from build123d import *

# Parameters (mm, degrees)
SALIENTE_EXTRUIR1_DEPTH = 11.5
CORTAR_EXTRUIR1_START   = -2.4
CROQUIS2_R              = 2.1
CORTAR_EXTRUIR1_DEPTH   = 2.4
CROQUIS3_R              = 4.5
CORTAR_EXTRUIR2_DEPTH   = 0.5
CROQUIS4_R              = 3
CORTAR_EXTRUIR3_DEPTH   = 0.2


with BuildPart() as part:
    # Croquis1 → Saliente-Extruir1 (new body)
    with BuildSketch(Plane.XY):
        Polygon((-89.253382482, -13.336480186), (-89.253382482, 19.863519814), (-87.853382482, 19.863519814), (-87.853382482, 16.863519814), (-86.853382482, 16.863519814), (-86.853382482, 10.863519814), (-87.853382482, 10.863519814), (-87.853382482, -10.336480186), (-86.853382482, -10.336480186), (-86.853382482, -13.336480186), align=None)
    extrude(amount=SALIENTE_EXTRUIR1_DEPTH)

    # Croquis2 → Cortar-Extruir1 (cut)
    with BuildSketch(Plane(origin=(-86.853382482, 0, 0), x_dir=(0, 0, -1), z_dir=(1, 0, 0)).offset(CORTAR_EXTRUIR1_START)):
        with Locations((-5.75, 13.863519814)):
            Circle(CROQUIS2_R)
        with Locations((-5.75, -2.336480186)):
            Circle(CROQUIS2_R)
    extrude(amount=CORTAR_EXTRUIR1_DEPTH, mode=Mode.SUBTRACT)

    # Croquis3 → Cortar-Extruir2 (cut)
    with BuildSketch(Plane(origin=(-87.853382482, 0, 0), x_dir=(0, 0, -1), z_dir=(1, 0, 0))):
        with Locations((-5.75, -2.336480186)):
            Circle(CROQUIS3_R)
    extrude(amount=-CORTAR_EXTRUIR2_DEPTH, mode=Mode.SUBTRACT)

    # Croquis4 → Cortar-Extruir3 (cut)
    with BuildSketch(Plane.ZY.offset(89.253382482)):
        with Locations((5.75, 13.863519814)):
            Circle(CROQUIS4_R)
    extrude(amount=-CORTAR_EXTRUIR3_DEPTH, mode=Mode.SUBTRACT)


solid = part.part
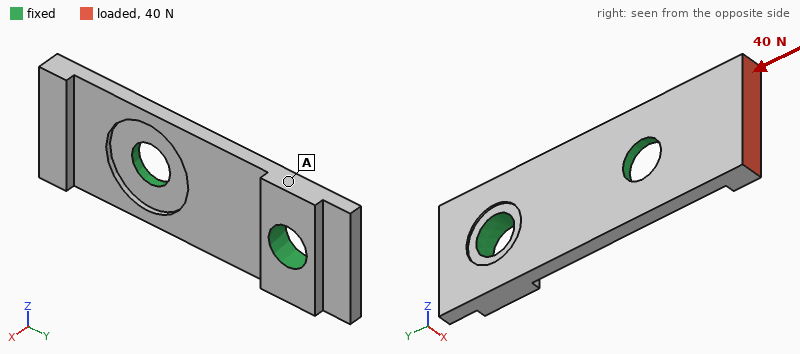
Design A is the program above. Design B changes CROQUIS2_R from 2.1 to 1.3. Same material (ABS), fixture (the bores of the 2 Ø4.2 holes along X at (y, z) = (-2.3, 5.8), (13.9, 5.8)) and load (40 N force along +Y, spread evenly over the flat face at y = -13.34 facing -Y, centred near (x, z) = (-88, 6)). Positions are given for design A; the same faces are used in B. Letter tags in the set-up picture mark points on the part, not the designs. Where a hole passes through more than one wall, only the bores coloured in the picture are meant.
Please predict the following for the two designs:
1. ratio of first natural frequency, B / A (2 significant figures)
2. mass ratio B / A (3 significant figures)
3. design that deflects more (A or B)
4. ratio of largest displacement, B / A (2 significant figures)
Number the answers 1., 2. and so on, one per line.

1. 0.81
2. 1.05
3. B
4. 1.3
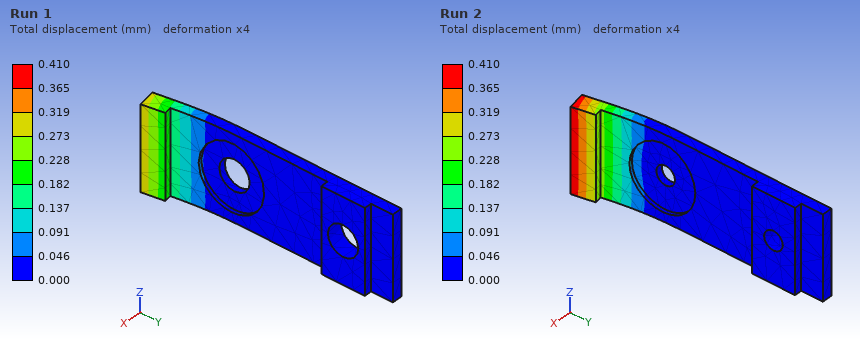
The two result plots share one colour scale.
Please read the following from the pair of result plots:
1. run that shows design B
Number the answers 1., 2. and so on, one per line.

1. Run 2
